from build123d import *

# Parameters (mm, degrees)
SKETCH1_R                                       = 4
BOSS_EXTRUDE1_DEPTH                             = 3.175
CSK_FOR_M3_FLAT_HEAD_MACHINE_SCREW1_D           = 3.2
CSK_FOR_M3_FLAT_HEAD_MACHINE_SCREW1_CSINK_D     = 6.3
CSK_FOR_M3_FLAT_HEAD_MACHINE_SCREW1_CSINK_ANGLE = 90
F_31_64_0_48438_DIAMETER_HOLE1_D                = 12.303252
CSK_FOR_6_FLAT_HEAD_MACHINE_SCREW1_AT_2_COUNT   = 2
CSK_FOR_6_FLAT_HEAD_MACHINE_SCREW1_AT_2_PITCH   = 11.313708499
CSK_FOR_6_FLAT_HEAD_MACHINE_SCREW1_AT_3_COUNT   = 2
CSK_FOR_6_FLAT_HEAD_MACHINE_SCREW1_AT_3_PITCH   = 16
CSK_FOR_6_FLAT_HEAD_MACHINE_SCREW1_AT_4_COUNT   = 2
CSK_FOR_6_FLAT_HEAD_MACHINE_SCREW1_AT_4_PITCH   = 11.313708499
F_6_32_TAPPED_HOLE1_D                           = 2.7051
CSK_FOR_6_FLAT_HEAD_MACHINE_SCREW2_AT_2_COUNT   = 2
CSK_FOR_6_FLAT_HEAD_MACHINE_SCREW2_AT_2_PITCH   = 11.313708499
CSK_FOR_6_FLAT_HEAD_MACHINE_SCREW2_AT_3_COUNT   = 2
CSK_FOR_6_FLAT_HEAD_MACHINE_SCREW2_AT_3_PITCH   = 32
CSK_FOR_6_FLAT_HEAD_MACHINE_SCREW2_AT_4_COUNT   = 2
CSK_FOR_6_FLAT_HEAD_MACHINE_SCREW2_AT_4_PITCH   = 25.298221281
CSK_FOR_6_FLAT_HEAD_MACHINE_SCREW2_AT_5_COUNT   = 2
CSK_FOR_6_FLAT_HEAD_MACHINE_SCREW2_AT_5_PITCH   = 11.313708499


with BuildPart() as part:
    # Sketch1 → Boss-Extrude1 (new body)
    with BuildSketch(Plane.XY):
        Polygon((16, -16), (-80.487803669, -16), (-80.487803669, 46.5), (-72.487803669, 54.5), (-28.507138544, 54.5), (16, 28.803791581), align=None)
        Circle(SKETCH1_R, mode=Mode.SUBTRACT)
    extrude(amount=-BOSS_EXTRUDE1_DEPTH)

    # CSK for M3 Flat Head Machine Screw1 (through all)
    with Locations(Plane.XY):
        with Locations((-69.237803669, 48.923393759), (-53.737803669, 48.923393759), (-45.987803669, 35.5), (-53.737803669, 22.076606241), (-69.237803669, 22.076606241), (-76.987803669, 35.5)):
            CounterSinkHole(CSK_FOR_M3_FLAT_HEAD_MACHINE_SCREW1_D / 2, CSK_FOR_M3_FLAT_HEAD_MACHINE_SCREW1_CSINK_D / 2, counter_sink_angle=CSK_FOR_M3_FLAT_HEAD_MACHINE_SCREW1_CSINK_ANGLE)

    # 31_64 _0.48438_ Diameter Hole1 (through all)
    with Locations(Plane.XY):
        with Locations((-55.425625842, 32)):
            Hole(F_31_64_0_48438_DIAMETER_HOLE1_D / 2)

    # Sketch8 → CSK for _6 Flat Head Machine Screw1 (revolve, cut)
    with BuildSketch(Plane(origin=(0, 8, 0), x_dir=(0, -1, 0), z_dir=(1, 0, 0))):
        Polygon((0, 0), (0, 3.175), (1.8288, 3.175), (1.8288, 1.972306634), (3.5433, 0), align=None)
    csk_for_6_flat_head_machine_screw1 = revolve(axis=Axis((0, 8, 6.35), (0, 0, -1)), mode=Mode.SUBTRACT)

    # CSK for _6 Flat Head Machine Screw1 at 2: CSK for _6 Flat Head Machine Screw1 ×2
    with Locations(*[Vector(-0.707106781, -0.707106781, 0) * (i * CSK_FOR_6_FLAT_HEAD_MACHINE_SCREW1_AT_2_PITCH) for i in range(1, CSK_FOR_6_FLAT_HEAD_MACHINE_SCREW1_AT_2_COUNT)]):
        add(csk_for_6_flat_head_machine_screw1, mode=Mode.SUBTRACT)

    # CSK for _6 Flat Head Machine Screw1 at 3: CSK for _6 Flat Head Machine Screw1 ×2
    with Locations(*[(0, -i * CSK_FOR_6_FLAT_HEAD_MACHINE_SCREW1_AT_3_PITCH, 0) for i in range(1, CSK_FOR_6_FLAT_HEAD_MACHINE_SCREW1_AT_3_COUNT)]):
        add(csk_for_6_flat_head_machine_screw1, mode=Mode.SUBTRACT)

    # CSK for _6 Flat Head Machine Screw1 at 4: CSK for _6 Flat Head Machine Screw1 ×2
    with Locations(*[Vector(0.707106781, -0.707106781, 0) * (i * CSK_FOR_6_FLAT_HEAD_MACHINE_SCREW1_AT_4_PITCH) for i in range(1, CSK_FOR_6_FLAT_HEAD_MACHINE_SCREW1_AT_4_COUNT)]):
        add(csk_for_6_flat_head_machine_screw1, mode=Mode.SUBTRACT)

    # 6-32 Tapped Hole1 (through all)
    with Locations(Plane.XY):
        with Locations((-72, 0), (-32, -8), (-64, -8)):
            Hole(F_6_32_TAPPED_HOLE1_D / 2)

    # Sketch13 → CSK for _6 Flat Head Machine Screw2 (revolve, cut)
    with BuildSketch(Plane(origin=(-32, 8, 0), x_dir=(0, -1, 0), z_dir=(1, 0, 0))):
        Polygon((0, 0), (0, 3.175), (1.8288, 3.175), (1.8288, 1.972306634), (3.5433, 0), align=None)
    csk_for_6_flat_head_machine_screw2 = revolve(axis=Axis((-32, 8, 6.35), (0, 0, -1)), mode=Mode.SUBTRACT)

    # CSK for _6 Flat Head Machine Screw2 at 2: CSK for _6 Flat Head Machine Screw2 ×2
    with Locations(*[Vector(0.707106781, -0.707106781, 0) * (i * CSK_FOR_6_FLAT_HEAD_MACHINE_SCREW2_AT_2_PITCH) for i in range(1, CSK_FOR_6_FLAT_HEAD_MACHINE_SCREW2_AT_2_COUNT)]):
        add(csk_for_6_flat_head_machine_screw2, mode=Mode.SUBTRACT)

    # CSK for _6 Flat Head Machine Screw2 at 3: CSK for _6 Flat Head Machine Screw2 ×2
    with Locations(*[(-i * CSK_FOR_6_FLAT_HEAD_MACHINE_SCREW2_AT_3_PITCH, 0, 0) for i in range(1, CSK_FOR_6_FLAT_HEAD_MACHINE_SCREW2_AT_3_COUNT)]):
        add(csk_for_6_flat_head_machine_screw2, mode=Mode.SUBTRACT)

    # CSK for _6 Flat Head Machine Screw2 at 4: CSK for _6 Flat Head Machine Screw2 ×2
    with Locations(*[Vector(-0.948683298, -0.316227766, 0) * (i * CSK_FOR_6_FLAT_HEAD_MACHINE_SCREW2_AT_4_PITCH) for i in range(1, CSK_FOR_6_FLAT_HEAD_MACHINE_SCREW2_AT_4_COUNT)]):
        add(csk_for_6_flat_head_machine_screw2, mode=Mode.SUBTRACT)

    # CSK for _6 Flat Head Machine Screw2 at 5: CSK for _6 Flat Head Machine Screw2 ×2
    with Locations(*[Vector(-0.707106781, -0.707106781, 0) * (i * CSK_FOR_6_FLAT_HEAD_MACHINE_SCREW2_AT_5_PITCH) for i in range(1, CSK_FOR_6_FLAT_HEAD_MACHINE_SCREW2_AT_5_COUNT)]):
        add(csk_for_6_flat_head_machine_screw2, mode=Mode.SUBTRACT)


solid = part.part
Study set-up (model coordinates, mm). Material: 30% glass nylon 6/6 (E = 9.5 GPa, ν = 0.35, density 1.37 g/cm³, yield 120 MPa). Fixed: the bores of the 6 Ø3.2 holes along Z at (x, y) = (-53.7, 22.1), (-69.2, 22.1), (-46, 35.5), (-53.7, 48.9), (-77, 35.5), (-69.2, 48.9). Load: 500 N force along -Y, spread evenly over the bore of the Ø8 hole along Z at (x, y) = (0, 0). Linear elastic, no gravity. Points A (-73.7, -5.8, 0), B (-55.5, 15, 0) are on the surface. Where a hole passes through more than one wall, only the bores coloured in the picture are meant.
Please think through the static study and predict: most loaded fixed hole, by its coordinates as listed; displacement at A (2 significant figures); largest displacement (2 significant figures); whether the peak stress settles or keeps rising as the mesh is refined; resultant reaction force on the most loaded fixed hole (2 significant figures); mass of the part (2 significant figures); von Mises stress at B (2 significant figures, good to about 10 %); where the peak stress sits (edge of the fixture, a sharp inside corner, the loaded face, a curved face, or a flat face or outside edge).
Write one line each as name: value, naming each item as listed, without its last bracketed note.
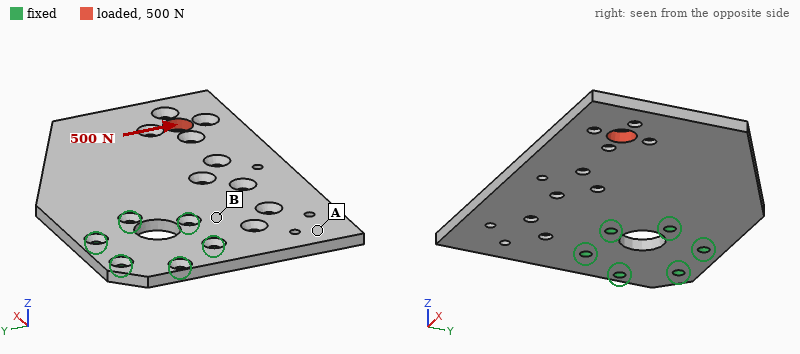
most loaded fixed hole, by its coordinates as listed: (-46, 35.5)
displacement at A: 0.063 mm
largest displacement: 0.22 mm
whether the peak stress settles or keeps rising as the mesh is refined: keeps rising
resultant reaction force on the most loaded fixed hole: 540 N
mass of the part: 25 g
von Mises stress at B: 9.7 MPa
where the peak stress sits: edge of the fixture
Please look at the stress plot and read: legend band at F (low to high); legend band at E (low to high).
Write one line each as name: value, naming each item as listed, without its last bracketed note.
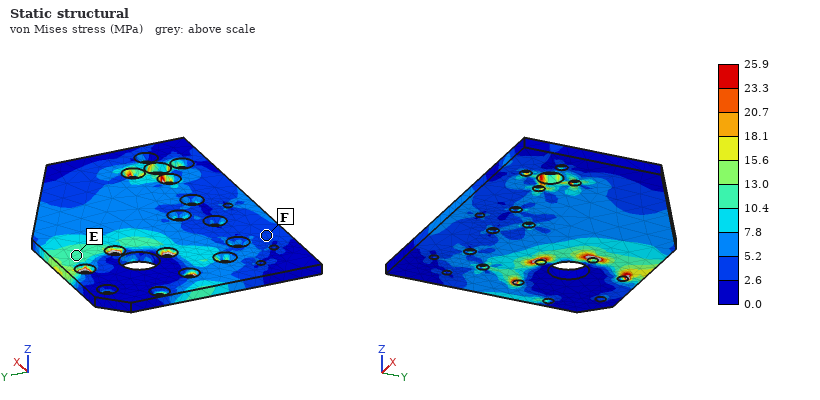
legend band at F: 2.6 to 5.2 MPa
legend band at E: 10.4 to 13.0 MPa
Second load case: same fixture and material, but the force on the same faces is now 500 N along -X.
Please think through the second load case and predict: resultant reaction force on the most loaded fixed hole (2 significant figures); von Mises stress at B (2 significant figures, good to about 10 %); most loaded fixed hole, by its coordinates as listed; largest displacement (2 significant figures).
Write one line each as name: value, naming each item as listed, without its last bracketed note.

resultant reaction force on the most loaded fixed hole: 400 N
von Mises stress at B: 9.0 MPa
most loaded fixed hole, by its coordinates as listed: (-53.7, 22.1)
largest displacement: 0.15 mm
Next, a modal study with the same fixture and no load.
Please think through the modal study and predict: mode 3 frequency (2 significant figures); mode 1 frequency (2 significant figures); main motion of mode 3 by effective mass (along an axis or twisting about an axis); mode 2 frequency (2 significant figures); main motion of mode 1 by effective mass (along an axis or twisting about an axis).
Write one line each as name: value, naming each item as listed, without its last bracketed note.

mode 3 frequency: 1100 Hz
mode 1 frequency: 290 Hz
main motion of mode 3 by effective mass: along Z
mode 2 frequency: 690 Hz
main motion of mode 1 by effective mass: along Z
